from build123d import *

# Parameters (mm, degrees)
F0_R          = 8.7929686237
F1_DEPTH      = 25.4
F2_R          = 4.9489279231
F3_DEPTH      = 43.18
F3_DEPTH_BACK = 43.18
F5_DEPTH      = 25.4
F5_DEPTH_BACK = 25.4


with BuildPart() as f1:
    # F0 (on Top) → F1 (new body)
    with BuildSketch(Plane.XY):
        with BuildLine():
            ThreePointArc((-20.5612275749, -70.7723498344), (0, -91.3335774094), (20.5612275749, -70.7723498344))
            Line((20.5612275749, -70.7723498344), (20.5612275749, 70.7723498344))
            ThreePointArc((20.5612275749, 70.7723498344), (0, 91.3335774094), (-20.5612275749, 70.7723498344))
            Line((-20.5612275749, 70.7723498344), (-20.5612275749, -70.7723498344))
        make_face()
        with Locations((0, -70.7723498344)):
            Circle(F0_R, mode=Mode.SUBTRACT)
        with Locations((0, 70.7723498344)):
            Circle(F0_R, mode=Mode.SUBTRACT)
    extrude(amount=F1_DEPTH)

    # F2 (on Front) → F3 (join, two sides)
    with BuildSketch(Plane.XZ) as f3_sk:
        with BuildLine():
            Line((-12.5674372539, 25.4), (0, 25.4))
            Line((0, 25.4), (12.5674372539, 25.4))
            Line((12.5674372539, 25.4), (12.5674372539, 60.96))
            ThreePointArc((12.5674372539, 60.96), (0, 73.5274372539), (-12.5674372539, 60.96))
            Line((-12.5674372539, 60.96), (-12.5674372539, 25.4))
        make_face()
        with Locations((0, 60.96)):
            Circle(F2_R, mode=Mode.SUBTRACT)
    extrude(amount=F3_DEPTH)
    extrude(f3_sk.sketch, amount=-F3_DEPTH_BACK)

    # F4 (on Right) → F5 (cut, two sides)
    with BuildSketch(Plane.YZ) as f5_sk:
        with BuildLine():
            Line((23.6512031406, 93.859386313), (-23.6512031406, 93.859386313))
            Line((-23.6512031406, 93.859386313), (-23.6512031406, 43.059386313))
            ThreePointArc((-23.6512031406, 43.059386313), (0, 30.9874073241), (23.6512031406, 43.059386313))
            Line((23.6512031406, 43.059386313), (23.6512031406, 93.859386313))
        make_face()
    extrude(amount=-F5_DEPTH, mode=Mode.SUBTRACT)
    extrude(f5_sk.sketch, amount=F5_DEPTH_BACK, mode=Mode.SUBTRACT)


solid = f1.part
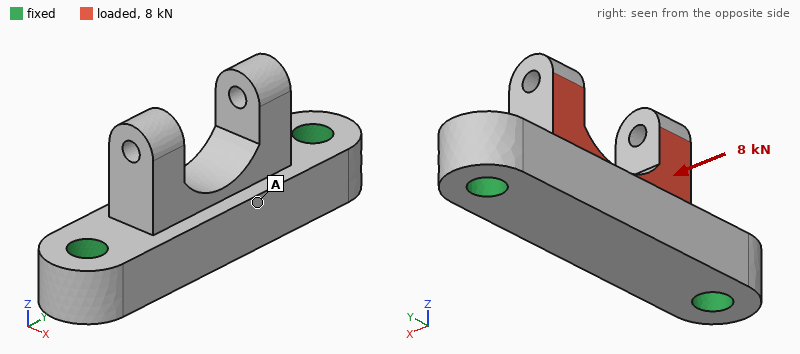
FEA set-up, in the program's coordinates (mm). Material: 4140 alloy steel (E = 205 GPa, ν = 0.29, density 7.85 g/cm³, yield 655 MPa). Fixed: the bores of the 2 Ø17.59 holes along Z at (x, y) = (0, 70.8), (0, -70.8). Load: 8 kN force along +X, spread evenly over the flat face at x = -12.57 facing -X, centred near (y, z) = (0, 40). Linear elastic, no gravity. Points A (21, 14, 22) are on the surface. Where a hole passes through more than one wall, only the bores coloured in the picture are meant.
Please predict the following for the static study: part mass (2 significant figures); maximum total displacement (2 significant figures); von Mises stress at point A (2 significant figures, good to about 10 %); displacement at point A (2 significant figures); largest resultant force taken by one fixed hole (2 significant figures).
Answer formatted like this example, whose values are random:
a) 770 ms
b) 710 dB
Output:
a) 1.7 kg
b) 29 µm
c) 7.5 MPa
d) 9.9 µm
e) 4.0 kN
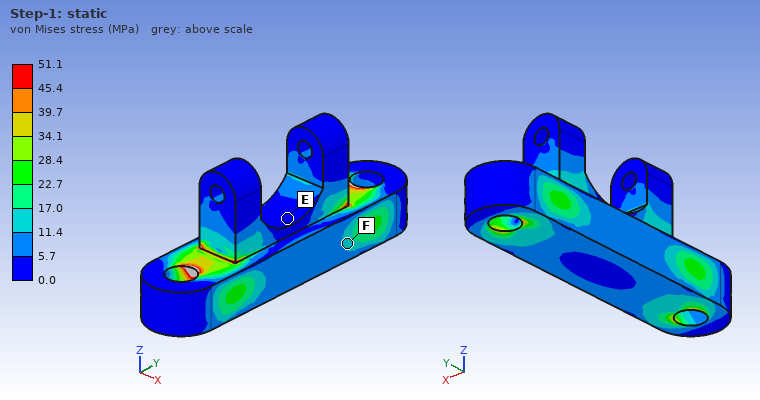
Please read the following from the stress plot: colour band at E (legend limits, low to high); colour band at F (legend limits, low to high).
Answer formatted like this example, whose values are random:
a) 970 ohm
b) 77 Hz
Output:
a) 0.0 to 5.7 MPa
b) 11.4 to 17.0 MPa
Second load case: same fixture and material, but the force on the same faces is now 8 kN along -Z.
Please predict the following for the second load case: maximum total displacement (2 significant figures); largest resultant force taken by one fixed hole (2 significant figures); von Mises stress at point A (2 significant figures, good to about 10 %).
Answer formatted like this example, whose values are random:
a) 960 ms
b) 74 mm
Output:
a) 16 µm
b) 4.1 kN
c) 4.3 MPa
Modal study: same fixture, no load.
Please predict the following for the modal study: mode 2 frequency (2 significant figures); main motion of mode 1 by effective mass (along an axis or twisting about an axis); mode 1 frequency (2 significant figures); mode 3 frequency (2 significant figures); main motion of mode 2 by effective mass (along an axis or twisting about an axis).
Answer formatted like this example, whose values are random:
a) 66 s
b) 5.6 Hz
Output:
a) 5400 Hz
b) along X
c) 4400 Hz
d) 6600 Hz
e) along Z
